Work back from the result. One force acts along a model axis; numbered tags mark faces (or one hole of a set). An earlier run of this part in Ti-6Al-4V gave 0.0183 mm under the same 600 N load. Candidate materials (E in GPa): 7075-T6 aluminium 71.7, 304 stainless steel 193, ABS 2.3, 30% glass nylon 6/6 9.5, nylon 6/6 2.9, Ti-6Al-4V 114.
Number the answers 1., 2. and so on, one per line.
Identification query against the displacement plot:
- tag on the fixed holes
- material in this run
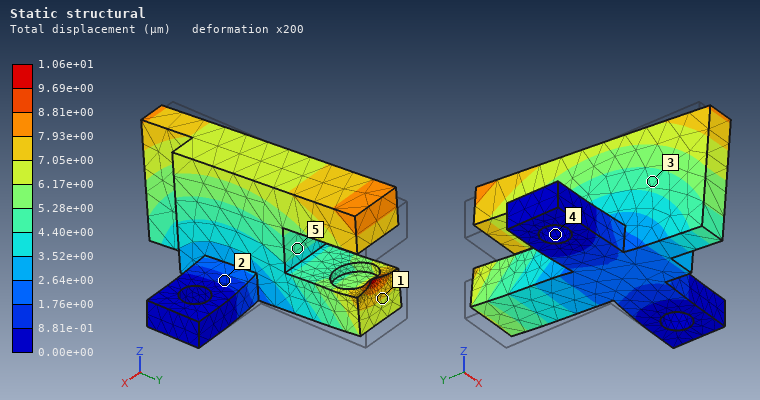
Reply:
1. 4
2. 304 stainless steel
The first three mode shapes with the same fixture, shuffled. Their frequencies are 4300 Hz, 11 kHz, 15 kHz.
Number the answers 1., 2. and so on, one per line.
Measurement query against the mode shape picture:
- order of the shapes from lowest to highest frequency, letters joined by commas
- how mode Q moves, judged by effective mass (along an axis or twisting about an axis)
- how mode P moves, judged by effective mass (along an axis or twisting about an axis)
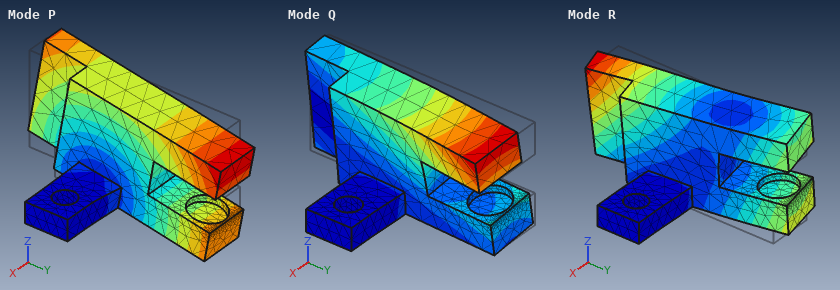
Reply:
1. P, Q, R
2. along X
3. along Y
